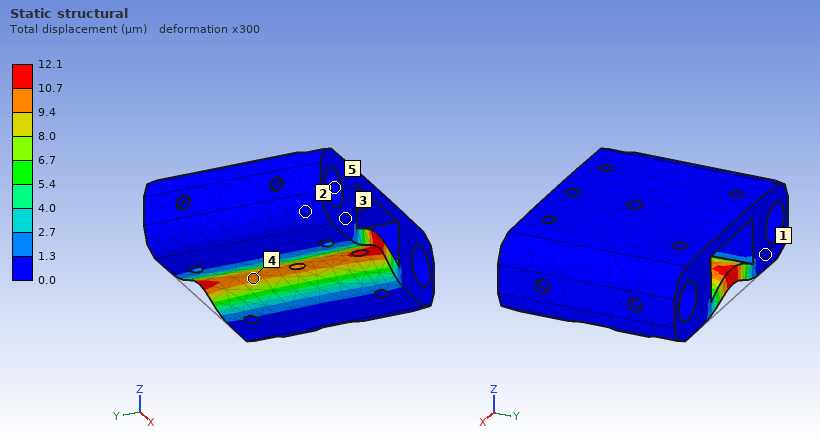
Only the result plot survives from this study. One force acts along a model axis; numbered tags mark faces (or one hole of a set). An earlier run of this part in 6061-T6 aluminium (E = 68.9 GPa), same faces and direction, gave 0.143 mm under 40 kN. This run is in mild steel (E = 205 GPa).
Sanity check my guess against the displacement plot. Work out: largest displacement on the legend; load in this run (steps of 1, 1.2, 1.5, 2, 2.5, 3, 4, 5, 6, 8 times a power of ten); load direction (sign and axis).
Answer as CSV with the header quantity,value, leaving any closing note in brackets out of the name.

quantity,value
largest displacement on the legend,12.1 µm
load in this run,10 kN
load direction,+Z
